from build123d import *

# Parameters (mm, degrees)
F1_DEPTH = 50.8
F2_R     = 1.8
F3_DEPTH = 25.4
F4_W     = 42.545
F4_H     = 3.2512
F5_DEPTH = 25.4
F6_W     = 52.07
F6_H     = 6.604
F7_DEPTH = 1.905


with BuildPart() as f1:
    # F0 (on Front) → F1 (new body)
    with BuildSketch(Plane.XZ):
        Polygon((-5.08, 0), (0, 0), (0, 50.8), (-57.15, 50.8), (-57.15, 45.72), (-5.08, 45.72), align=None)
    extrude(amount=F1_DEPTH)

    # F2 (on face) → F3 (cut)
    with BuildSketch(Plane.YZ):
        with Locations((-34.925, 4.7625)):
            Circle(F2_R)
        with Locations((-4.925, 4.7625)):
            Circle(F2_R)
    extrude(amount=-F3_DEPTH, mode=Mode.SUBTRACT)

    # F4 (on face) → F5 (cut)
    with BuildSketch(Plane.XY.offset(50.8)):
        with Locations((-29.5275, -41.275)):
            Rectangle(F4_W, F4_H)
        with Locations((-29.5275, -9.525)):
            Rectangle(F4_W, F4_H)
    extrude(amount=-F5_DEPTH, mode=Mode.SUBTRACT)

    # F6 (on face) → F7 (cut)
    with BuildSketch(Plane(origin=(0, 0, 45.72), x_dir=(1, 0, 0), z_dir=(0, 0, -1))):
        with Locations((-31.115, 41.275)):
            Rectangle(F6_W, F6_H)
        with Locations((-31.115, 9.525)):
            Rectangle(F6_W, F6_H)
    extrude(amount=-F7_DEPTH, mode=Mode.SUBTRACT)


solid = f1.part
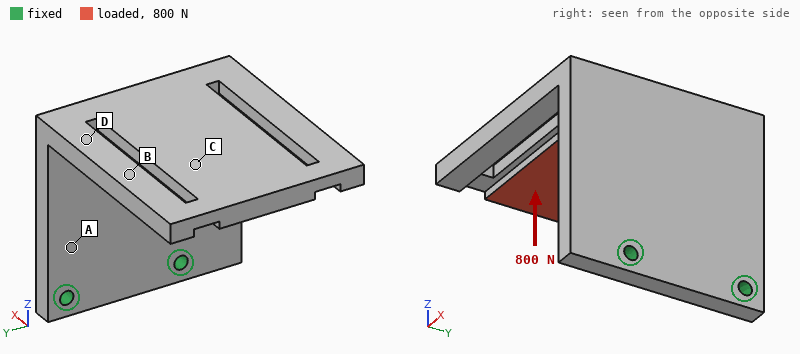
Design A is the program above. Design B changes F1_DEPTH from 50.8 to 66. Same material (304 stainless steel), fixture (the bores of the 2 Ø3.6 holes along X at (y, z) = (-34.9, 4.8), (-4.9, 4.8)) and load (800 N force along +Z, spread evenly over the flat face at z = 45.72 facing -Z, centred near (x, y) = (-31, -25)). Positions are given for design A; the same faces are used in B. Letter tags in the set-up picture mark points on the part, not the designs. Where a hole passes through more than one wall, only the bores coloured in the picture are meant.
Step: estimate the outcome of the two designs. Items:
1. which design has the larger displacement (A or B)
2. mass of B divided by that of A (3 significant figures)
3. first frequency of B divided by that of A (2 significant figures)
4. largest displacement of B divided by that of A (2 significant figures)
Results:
A
1.33
0.92
0.84
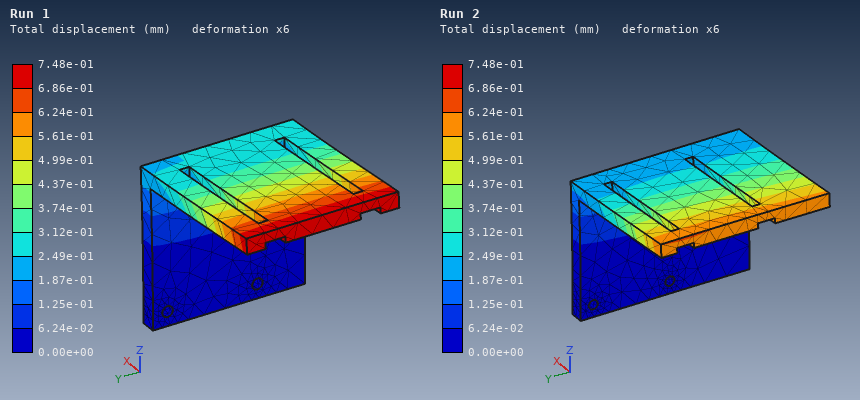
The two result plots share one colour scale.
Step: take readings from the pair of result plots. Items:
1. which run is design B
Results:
Run 2
